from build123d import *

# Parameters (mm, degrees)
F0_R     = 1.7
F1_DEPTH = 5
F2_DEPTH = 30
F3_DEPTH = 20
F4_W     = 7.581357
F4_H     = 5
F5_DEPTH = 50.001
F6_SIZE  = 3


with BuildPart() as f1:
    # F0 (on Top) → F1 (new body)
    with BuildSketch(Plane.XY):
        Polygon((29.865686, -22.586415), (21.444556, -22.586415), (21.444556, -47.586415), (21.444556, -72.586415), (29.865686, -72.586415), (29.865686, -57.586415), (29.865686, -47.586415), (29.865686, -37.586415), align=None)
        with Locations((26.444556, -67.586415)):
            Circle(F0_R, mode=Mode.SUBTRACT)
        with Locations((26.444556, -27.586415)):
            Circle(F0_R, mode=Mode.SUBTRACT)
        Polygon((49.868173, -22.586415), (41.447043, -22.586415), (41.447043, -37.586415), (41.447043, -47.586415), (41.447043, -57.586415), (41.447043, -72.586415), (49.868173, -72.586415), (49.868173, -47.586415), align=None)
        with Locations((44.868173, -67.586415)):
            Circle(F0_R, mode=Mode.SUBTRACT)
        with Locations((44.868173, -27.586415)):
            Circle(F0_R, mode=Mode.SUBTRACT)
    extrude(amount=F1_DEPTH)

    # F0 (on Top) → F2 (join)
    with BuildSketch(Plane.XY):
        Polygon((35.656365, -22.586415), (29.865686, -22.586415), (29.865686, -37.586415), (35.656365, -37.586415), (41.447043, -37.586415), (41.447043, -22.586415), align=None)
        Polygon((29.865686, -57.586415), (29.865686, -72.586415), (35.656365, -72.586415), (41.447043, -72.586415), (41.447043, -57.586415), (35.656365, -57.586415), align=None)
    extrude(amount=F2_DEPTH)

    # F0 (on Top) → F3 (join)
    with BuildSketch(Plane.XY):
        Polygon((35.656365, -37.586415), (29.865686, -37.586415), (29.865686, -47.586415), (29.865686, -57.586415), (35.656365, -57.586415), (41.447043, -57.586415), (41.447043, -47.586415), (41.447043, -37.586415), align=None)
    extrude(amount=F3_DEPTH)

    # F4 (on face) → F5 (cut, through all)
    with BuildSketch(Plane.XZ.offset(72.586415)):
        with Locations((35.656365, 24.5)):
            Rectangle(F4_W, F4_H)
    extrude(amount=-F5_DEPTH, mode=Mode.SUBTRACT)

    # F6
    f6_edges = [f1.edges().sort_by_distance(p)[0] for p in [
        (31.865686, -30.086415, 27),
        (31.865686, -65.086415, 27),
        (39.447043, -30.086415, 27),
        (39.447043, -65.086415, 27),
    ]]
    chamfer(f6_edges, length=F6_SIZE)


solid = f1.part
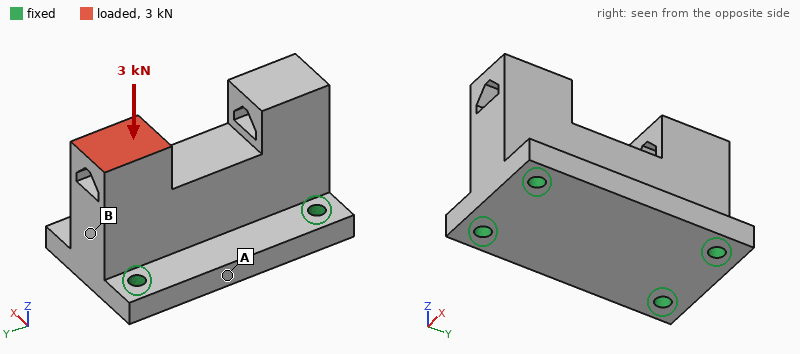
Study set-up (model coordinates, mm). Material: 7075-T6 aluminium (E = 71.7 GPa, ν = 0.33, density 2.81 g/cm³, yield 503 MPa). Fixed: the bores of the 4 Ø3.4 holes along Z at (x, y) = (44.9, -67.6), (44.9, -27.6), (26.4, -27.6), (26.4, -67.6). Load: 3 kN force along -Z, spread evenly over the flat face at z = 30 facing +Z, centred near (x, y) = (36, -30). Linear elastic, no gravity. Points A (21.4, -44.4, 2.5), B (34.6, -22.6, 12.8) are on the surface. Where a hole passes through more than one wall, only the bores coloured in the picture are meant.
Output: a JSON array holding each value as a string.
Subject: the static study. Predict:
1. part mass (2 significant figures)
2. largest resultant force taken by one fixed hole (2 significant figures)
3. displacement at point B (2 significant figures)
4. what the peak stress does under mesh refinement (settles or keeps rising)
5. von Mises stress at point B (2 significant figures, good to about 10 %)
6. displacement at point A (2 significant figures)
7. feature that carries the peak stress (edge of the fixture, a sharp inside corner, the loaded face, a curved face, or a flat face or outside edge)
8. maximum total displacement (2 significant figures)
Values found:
["51 g", "1.5 kN", "9.4 µm", "keeps rising", "16 MPa", "4.2 µm", "edge of the fixture", "22 µm"]
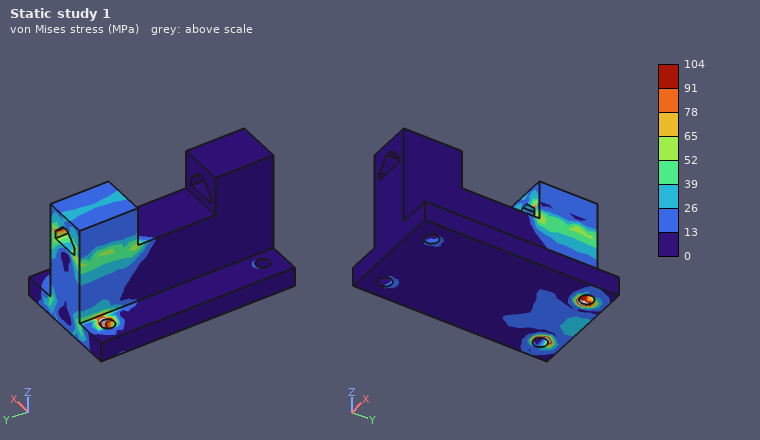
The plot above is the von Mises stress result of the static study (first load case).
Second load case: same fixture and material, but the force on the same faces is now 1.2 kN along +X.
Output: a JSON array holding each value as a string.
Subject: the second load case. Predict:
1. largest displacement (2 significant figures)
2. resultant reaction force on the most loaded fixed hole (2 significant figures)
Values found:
["78 µm", "1.6 kN"]
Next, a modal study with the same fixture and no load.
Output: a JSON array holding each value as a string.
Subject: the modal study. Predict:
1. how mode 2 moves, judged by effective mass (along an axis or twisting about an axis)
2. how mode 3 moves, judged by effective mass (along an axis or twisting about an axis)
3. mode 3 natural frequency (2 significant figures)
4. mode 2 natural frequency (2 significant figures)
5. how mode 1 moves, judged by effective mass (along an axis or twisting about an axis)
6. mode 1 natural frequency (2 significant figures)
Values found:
["twisting about Z", "along Z", "17 kHz", "13 kHz", "along X", "9700 Hz"]
